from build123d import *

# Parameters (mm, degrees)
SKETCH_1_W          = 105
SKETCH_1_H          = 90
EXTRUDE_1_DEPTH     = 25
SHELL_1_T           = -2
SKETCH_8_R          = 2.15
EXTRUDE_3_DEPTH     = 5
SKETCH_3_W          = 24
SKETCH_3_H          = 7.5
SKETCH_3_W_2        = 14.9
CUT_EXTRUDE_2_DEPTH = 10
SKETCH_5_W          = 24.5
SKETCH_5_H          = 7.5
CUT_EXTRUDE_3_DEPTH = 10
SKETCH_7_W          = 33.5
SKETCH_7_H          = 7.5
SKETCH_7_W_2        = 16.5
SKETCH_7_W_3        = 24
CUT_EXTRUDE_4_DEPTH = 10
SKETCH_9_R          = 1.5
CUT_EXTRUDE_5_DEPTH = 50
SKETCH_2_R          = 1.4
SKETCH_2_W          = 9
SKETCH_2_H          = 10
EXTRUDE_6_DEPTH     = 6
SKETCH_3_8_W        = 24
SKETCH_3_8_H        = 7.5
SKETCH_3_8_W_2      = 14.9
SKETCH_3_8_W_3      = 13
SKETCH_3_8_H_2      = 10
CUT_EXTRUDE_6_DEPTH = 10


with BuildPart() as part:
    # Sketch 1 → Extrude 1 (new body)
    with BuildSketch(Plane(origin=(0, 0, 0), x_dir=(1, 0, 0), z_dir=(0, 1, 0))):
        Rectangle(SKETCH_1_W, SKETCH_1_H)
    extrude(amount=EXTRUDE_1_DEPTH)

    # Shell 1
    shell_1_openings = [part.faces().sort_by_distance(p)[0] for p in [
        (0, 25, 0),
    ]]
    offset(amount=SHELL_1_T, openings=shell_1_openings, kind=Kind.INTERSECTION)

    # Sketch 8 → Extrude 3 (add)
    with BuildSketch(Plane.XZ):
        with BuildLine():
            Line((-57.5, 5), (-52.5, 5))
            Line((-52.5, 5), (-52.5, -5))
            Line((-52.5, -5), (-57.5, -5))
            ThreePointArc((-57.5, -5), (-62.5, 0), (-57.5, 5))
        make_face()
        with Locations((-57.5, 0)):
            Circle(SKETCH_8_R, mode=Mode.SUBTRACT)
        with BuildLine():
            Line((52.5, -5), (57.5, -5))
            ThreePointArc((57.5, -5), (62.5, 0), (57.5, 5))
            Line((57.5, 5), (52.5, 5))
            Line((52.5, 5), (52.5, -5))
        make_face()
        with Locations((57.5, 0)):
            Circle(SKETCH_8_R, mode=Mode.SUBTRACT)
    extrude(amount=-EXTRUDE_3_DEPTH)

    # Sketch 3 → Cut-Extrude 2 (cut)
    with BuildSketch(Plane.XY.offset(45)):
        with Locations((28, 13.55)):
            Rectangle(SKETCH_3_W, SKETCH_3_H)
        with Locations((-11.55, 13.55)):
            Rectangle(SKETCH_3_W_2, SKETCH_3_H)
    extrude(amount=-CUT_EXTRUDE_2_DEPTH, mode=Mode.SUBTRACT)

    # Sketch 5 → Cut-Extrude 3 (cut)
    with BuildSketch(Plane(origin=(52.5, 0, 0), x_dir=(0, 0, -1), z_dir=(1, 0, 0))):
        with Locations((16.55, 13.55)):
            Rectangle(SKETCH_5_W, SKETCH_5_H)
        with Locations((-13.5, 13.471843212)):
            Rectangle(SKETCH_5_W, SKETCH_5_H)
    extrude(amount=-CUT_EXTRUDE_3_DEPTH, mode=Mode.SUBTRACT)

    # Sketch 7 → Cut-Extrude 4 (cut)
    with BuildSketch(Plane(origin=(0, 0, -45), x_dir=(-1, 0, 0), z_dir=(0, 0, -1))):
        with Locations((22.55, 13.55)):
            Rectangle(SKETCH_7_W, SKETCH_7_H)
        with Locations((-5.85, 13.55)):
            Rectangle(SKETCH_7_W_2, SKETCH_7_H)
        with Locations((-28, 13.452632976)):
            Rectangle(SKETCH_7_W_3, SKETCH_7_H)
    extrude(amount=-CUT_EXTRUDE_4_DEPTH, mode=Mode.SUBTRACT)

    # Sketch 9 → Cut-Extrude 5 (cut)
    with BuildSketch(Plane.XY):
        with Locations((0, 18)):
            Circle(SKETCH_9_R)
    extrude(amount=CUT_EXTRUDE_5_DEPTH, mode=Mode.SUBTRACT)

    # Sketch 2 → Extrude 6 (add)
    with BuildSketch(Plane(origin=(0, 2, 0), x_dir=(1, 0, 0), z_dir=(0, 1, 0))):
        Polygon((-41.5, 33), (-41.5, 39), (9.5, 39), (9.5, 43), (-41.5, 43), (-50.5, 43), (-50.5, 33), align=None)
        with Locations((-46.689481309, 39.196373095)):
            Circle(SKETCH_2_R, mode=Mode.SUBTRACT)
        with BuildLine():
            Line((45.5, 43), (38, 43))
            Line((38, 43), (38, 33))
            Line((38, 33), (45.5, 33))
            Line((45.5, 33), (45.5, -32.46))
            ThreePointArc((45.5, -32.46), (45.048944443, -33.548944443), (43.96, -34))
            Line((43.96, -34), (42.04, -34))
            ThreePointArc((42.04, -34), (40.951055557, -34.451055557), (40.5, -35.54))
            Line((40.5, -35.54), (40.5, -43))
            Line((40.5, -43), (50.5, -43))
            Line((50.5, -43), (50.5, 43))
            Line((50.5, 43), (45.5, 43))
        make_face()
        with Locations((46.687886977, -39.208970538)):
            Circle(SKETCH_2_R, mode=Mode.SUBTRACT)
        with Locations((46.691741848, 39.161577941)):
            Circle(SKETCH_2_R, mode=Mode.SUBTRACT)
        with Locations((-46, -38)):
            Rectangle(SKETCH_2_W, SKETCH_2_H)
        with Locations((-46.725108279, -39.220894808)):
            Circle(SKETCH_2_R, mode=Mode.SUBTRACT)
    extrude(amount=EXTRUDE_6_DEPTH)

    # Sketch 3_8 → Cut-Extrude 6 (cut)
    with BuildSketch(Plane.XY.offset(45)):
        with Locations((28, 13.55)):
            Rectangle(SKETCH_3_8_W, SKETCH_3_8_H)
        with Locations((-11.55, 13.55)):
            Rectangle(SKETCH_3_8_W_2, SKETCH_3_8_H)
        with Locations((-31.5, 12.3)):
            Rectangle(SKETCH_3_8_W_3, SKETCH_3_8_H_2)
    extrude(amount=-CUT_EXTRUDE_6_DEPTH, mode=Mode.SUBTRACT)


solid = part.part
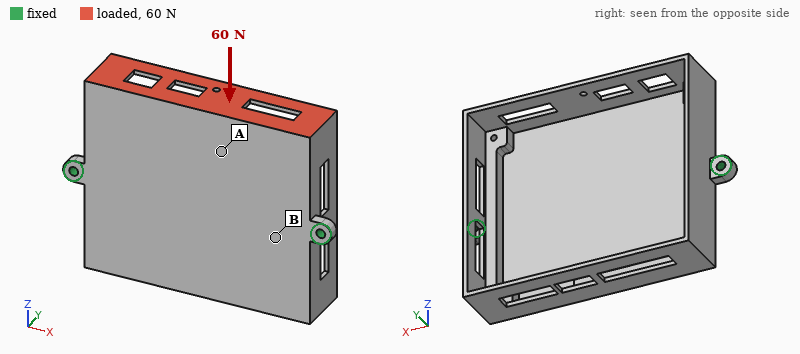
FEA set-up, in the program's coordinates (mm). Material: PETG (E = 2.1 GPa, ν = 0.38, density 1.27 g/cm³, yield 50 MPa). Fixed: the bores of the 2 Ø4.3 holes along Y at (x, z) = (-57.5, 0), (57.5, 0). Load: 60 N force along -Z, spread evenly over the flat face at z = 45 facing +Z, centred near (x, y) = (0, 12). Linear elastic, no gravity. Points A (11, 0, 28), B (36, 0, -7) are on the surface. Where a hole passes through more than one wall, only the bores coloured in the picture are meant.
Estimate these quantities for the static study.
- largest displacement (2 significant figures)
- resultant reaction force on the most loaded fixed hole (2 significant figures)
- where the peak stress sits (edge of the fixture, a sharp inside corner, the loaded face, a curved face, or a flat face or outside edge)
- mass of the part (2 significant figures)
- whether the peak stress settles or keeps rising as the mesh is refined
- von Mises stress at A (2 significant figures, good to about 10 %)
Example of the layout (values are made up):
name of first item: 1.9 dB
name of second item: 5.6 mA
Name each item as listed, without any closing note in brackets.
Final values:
largest displacement: 1.5 mm
resultant reaction force on the most loaded fixed hole: 30 N
where the peak stress sits: edge of the fixture
mass of the part: 51 g
whether the peak stress settles or keeps rising as the mesh is refined: keeps rising
von Mises stress at A: 2.0 MPa
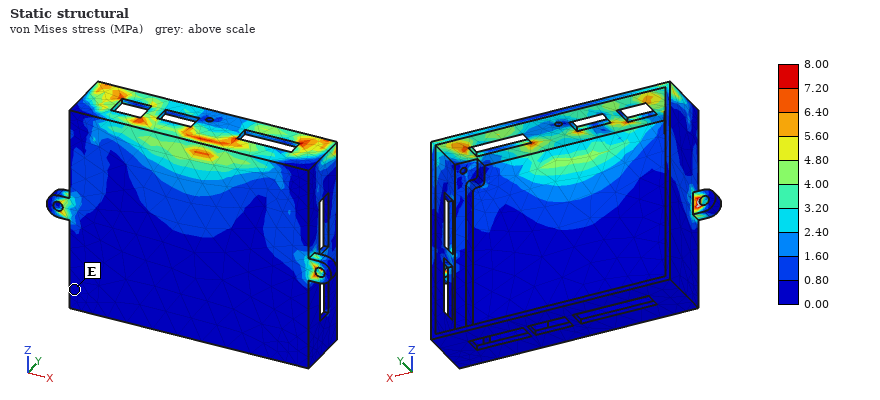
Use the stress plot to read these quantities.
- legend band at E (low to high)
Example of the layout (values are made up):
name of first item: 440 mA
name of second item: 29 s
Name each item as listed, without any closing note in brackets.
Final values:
legend band at E: 0.00 to 0.80 MPa
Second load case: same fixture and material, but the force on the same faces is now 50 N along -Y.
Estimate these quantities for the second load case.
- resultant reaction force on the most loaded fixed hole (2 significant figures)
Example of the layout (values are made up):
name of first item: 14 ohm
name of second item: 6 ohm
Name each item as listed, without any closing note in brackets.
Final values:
resultant reaction force on the most loaded fixed hole: 26 N
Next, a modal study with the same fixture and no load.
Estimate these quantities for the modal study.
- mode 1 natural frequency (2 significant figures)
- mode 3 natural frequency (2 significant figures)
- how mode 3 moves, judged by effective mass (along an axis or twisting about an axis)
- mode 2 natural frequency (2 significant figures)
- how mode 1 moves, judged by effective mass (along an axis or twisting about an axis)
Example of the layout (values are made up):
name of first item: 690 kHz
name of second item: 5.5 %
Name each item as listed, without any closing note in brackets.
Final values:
mode 1 natural frequency: 200 Hz
mode 3 natural frequency: 410 Hz
how mode 3 moves, judged by effective mass: along Y
mode 2 natural frequency: 330 Hz
how mode 1 moves, judged by effective mass: twisting about X
